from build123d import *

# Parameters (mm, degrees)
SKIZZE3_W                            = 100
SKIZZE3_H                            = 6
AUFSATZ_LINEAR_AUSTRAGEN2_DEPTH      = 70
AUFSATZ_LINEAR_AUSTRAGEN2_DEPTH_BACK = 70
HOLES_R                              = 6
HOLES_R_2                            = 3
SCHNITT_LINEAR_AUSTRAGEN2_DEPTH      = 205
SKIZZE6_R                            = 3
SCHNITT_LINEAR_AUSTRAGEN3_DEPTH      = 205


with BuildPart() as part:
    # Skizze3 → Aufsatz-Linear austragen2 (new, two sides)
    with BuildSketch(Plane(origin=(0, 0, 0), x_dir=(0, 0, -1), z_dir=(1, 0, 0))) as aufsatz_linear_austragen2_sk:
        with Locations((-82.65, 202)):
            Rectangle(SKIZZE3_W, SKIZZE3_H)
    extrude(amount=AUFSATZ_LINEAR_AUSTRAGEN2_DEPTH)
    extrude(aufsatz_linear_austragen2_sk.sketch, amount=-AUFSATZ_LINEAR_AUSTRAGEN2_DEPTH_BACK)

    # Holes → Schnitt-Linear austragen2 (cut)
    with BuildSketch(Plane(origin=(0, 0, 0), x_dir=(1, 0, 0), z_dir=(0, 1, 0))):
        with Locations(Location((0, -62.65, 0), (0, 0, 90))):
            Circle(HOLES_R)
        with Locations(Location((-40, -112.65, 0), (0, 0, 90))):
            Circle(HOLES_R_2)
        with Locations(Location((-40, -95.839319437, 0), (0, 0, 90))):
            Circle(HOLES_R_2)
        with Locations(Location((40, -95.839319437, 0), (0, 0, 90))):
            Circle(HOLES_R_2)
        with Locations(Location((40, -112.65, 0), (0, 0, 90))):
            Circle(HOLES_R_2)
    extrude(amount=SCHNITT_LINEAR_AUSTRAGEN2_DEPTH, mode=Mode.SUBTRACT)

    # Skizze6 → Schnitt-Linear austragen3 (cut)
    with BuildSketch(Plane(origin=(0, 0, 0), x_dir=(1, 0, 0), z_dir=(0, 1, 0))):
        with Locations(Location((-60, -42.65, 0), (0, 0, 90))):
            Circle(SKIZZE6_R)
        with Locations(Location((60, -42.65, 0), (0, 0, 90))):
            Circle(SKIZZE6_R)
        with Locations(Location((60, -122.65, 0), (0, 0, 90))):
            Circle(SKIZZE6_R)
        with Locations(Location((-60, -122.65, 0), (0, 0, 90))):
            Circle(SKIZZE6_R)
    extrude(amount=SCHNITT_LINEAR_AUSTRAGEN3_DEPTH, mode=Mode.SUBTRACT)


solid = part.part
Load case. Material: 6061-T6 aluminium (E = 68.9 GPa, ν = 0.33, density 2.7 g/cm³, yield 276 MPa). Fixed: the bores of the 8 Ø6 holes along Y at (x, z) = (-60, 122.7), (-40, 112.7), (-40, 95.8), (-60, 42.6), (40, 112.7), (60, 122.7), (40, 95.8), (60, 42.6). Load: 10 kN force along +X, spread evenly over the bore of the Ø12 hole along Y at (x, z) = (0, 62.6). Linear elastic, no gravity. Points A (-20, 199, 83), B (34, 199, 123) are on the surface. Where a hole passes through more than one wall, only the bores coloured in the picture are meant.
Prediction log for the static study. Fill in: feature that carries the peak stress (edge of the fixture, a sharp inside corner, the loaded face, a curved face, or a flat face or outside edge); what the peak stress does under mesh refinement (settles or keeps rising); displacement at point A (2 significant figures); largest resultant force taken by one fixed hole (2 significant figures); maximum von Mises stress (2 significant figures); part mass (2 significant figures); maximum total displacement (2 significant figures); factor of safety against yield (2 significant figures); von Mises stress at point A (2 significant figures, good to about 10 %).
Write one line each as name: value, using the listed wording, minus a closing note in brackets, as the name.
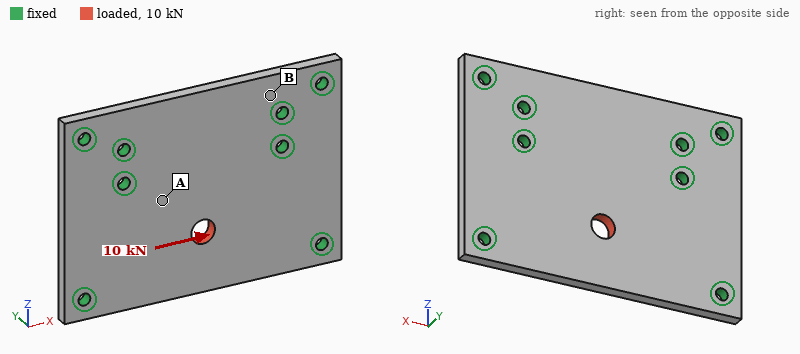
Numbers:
feature that carries the peak stress: the loaded face
what the peak stress does under mesh refinement: settles
displacement at point A: 5.8 µm
largest resultant force taken by one fixed hole: 2.5 kN
maximum von Mises stress: 77 MPa
part mass: 220 g
maximum total displacement: 19 µm
factor of safety against yield: 3.6
von Mises stress at point A: 16 MPa
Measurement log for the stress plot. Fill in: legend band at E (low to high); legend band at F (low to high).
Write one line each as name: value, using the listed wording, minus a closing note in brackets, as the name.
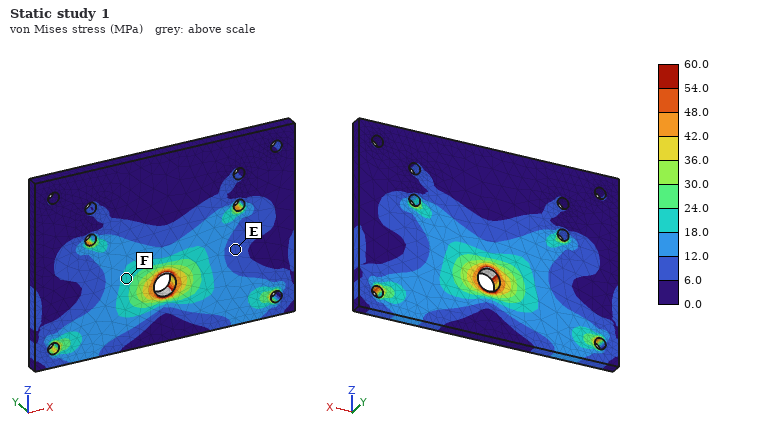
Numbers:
legend band at E: 6.0 to 12.0 MPa
legend band at F: 18.0 to 24.0 MPa
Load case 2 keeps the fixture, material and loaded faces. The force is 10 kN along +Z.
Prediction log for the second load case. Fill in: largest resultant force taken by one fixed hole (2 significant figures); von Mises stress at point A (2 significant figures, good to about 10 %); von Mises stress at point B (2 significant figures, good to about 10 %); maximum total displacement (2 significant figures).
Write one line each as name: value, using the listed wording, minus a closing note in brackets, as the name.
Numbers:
largest resultant force taken by one fixed hole: 2.7 kN
von Mises stress at point A: 23 MPa
von Mises stress at point B: 10 MPa
maximum total displacement: 28 µm
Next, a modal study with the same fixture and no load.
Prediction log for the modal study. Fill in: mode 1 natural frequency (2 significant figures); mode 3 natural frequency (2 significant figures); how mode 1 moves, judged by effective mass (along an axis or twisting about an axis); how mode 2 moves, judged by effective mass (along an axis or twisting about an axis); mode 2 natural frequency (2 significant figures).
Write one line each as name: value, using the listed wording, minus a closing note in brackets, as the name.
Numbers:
mode 1 natural frequency: 2600 Hz
mode 3 natural frequency: 6100 Hz
how mode 1 moves, judged by effective mass: along Y
how mode 2 moves, judged by effective mass: along Y
mode 2 natural frequency: 4800 Hz
